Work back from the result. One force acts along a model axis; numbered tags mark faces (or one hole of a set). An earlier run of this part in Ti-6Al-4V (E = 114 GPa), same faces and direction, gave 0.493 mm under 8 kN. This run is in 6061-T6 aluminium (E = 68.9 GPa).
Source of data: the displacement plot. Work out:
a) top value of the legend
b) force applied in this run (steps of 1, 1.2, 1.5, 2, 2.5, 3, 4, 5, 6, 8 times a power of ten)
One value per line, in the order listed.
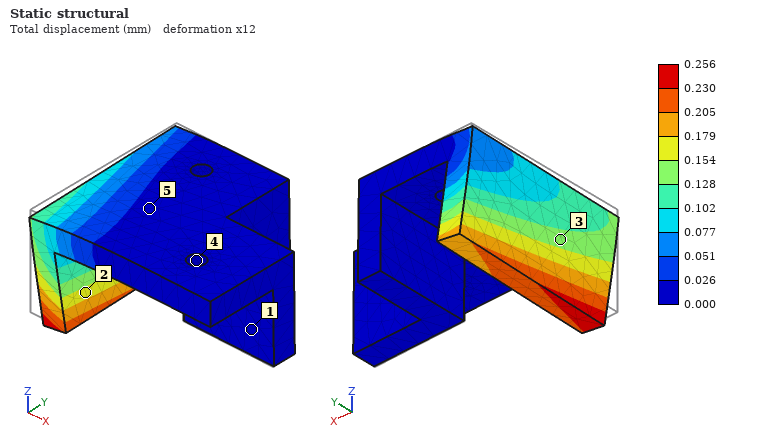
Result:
0.256 mm
2.5 kN
